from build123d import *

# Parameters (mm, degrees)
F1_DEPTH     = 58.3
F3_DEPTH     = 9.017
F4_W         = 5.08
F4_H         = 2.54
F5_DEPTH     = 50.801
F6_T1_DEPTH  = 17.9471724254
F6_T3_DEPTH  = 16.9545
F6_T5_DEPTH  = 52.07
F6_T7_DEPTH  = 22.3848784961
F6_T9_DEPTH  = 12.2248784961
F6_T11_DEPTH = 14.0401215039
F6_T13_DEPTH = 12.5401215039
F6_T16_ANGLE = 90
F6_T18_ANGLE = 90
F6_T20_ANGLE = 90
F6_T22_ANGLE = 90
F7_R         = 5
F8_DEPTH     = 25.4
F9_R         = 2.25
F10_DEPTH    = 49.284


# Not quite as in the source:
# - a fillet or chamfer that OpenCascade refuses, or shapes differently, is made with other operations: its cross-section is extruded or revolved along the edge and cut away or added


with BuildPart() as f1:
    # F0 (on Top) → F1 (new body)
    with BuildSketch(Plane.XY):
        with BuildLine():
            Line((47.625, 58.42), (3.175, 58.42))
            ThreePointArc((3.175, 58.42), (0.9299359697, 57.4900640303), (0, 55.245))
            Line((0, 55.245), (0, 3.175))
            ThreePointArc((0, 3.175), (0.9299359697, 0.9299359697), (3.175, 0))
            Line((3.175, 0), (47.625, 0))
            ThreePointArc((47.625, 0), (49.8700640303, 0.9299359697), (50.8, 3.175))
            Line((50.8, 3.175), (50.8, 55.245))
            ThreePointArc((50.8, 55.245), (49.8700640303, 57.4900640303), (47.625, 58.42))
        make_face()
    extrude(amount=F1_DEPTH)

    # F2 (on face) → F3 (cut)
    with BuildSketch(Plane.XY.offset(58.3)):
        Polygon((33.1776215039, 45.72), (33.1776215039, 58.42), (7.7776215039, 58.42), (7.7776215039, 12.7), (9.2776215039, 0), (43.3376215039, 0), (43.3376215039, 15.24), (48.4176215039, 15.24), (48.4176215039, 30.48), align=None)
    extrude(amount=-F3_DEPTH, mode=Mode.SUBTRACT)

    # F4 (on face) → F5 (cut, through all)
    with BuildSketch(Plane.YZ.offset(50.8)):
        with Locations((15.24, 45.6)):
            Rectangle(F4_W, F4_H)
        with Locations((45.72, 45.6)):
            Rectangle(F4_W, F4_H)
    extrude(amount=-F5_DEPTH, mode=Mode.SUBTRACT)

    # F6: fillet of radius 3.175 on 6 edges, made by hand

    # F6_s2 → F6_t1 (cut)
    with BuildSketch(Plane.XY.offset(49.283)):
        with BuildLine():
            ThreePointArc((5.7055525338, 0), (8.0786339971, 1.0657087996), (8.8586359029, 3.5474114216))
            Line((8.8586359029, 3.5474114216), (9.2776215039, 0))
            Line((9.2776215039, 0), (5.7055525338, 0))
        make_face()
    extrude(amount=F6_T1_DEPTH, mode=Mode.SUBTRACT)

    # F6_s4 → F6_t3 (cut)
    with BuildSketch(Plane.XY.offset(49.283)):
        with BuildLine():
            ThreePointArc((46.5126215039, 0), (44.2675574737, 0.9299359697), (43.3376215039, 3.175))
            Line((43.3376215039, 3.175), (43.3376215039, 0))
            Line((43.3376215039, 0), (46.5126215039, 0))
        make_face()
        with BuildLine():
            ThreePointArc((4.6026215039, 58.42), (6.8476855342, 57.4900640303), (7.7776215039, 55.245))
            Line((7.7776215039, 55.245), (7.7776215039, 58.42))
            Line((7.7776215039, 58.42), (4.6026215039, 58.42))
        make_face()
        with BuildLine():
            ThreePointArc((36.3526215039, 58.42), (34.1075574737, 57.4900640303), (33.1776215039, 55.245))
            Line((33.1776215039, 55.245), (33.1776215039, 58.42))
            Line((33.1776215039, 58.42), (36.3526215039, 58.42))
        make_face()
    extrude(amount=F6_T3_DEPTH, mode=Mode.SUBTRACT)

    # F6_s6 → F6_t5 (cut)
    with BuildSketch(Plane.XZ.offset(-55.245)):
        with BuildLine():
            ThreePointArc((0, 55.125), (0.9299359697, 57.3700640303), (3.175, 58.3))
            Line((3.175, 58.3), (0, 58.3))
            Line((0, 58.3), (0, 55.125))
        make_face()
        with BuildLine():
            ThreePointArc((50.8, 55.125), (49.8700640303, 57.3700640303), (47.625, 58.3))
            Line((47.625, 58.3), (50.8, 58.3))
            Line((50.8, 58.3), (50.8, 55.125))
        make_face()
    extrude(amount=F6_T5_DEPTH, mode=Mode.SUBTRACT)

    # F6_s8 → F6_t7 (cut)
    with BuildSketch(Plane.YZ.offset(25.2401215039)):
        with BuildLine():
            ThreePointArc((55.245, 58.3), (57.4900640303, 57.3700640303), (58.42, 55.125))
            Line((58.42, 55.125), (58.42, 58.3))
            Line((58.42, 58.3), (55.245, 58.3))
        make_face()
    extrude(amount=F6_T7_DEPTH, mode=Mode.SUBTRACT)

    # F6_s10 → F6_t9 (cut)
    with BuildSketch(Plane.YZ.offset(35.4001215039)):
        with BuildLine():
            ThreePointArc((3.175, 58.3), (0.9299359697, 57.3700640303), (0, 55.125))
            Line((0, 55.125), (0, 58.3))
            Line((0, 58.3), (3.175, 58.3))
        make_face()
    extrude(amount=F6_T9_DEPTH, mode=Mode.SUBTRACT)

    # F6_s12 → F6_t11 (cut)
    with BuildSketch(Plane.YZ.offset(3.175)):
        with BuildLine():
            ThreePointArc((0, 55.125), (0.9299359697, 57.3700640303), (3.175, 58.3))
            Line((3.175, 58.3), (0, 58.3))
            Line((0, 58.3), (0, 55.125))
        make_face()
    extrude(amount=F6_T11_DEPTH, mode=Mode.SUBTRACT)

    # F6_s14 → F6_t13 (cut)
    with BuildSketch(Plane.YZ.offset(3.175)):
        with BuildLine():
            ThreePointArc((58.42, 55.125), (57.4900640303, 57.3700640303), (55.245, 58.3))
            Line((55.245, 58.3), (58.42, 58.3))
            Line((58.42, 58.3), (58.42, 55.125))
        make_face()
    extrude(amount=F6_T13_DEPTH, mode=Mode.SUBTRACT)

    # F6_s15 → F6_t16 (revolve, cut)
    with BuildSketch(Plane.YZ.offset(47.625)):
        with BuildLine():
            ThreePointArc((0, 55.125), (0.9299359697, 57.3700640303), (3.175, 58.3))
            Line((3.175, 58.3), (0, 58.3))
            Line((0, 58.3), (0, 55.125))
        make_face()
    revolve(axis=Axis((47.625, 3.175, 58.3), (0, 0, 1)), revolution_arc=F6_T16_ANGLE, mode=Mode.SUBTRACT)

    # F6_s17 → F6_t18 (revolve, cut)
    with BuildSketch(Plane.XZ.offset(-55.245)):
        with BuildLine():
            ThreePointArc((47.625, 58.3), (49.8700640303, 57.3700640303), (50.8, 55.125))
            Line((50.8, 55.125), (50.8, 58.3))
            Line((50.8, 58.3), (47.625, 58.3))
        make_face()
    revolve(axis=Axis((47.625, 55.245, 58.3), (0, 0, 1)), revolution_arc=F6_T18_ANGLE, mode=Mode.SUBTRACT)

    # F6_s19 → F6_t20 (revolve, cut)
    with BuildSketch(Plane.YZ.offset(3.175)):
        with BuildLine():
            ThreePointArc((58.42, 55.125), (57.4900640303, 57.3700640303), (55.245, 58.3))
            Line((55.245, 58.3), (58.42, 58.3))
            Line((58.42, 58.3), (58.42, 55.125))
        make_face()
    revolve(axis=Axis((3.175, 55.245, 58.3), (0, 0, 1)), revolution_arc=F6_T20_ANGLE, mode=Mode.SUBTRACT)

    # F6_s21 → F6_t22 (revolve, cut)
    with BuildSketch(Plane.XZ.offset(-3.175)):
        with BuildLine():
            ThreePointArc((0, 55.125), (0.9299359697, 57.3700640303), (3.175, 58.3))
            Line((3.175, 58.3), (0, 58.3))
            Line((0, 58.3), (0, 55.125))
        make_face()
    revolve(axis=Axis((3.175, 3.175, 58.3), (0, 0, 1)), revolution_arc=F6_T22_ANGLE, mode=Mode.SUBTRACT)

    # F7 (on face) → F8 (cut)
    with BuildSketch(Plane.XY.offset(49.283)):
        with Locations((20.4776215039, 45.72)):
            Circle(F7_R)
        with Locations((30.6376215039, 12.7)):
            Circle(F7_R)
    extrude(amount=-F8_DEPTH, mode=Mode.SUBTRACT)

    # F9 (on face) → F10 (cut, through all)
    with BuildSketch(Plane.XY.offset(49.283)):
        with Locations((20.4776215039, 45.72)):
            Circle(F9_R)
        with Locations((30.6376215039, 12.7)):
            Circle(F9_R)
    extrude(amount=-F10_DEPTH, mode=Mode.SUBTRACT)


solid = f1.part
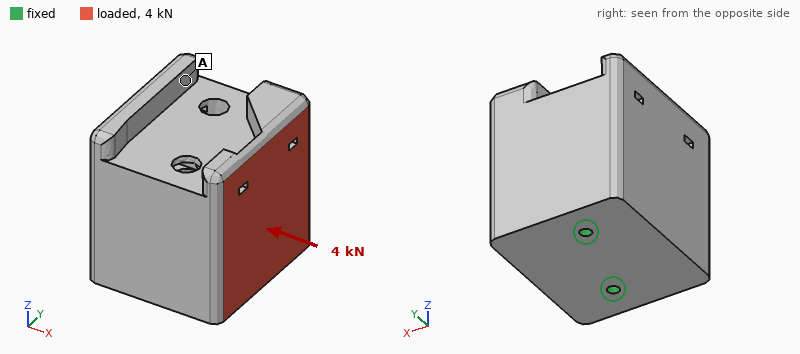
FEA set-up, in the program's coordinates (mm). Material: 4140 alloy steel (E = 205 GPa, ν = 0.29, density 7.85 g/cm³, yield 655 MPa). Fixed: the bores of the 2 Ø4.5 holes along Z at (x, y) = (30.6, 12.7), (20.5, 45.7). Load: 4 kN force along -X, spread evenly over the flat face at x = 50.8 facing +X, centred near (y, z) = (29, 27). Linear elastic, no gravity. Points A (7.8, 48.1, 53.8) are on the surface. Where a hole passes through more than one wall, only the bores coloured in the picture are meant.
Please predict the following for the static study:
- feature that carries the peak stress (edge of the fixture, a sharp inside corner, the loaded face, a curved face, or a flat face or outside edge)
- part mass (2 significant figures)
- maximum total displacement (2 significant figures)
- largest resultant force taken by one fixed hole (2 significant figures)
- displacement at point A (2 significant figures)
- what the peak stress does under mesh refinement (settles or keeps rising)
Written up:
edge of the fixture
1.2 kg
4.4 µm
2.0 kN
2.5 µm
keeps rising
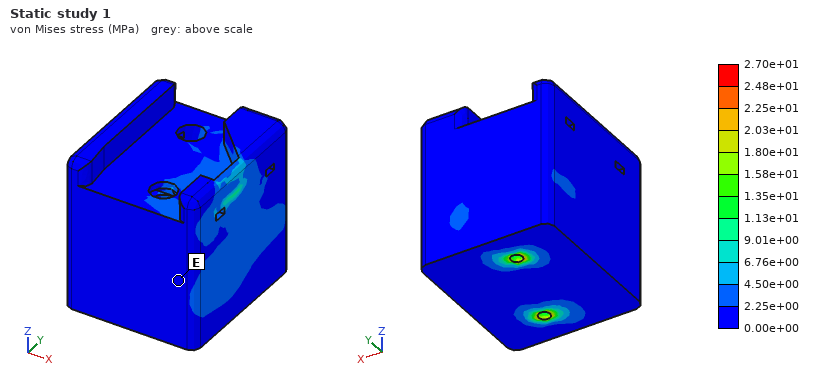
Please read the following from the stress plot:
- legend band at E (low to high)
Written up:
0.00e+00 to 2.25e+00 MPa
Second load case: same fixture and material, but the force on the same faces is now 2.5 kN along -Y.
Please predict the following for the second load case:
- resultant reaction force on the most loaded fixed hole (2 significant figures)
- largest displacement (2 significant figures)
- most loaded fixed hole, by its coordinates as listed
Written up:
2.5 kN
1.8 µm
(30.6, 12.7)
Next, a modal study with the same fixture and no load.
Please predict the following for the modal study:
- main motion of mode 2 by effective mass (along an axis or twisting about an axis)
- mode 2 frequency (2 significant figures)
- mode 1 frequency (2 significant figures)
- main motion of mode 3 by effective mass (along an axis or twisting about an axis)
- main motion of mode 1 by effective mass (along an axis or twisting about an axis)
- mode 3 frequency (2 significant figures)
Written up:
along Y
10 kHz
6000 Hz
twisting about Z
along X
13 kHz
